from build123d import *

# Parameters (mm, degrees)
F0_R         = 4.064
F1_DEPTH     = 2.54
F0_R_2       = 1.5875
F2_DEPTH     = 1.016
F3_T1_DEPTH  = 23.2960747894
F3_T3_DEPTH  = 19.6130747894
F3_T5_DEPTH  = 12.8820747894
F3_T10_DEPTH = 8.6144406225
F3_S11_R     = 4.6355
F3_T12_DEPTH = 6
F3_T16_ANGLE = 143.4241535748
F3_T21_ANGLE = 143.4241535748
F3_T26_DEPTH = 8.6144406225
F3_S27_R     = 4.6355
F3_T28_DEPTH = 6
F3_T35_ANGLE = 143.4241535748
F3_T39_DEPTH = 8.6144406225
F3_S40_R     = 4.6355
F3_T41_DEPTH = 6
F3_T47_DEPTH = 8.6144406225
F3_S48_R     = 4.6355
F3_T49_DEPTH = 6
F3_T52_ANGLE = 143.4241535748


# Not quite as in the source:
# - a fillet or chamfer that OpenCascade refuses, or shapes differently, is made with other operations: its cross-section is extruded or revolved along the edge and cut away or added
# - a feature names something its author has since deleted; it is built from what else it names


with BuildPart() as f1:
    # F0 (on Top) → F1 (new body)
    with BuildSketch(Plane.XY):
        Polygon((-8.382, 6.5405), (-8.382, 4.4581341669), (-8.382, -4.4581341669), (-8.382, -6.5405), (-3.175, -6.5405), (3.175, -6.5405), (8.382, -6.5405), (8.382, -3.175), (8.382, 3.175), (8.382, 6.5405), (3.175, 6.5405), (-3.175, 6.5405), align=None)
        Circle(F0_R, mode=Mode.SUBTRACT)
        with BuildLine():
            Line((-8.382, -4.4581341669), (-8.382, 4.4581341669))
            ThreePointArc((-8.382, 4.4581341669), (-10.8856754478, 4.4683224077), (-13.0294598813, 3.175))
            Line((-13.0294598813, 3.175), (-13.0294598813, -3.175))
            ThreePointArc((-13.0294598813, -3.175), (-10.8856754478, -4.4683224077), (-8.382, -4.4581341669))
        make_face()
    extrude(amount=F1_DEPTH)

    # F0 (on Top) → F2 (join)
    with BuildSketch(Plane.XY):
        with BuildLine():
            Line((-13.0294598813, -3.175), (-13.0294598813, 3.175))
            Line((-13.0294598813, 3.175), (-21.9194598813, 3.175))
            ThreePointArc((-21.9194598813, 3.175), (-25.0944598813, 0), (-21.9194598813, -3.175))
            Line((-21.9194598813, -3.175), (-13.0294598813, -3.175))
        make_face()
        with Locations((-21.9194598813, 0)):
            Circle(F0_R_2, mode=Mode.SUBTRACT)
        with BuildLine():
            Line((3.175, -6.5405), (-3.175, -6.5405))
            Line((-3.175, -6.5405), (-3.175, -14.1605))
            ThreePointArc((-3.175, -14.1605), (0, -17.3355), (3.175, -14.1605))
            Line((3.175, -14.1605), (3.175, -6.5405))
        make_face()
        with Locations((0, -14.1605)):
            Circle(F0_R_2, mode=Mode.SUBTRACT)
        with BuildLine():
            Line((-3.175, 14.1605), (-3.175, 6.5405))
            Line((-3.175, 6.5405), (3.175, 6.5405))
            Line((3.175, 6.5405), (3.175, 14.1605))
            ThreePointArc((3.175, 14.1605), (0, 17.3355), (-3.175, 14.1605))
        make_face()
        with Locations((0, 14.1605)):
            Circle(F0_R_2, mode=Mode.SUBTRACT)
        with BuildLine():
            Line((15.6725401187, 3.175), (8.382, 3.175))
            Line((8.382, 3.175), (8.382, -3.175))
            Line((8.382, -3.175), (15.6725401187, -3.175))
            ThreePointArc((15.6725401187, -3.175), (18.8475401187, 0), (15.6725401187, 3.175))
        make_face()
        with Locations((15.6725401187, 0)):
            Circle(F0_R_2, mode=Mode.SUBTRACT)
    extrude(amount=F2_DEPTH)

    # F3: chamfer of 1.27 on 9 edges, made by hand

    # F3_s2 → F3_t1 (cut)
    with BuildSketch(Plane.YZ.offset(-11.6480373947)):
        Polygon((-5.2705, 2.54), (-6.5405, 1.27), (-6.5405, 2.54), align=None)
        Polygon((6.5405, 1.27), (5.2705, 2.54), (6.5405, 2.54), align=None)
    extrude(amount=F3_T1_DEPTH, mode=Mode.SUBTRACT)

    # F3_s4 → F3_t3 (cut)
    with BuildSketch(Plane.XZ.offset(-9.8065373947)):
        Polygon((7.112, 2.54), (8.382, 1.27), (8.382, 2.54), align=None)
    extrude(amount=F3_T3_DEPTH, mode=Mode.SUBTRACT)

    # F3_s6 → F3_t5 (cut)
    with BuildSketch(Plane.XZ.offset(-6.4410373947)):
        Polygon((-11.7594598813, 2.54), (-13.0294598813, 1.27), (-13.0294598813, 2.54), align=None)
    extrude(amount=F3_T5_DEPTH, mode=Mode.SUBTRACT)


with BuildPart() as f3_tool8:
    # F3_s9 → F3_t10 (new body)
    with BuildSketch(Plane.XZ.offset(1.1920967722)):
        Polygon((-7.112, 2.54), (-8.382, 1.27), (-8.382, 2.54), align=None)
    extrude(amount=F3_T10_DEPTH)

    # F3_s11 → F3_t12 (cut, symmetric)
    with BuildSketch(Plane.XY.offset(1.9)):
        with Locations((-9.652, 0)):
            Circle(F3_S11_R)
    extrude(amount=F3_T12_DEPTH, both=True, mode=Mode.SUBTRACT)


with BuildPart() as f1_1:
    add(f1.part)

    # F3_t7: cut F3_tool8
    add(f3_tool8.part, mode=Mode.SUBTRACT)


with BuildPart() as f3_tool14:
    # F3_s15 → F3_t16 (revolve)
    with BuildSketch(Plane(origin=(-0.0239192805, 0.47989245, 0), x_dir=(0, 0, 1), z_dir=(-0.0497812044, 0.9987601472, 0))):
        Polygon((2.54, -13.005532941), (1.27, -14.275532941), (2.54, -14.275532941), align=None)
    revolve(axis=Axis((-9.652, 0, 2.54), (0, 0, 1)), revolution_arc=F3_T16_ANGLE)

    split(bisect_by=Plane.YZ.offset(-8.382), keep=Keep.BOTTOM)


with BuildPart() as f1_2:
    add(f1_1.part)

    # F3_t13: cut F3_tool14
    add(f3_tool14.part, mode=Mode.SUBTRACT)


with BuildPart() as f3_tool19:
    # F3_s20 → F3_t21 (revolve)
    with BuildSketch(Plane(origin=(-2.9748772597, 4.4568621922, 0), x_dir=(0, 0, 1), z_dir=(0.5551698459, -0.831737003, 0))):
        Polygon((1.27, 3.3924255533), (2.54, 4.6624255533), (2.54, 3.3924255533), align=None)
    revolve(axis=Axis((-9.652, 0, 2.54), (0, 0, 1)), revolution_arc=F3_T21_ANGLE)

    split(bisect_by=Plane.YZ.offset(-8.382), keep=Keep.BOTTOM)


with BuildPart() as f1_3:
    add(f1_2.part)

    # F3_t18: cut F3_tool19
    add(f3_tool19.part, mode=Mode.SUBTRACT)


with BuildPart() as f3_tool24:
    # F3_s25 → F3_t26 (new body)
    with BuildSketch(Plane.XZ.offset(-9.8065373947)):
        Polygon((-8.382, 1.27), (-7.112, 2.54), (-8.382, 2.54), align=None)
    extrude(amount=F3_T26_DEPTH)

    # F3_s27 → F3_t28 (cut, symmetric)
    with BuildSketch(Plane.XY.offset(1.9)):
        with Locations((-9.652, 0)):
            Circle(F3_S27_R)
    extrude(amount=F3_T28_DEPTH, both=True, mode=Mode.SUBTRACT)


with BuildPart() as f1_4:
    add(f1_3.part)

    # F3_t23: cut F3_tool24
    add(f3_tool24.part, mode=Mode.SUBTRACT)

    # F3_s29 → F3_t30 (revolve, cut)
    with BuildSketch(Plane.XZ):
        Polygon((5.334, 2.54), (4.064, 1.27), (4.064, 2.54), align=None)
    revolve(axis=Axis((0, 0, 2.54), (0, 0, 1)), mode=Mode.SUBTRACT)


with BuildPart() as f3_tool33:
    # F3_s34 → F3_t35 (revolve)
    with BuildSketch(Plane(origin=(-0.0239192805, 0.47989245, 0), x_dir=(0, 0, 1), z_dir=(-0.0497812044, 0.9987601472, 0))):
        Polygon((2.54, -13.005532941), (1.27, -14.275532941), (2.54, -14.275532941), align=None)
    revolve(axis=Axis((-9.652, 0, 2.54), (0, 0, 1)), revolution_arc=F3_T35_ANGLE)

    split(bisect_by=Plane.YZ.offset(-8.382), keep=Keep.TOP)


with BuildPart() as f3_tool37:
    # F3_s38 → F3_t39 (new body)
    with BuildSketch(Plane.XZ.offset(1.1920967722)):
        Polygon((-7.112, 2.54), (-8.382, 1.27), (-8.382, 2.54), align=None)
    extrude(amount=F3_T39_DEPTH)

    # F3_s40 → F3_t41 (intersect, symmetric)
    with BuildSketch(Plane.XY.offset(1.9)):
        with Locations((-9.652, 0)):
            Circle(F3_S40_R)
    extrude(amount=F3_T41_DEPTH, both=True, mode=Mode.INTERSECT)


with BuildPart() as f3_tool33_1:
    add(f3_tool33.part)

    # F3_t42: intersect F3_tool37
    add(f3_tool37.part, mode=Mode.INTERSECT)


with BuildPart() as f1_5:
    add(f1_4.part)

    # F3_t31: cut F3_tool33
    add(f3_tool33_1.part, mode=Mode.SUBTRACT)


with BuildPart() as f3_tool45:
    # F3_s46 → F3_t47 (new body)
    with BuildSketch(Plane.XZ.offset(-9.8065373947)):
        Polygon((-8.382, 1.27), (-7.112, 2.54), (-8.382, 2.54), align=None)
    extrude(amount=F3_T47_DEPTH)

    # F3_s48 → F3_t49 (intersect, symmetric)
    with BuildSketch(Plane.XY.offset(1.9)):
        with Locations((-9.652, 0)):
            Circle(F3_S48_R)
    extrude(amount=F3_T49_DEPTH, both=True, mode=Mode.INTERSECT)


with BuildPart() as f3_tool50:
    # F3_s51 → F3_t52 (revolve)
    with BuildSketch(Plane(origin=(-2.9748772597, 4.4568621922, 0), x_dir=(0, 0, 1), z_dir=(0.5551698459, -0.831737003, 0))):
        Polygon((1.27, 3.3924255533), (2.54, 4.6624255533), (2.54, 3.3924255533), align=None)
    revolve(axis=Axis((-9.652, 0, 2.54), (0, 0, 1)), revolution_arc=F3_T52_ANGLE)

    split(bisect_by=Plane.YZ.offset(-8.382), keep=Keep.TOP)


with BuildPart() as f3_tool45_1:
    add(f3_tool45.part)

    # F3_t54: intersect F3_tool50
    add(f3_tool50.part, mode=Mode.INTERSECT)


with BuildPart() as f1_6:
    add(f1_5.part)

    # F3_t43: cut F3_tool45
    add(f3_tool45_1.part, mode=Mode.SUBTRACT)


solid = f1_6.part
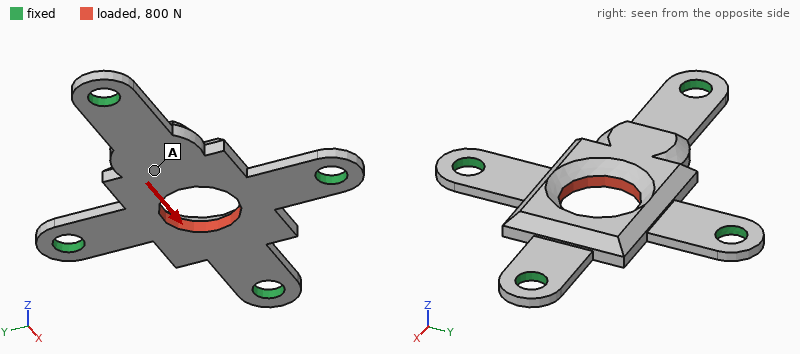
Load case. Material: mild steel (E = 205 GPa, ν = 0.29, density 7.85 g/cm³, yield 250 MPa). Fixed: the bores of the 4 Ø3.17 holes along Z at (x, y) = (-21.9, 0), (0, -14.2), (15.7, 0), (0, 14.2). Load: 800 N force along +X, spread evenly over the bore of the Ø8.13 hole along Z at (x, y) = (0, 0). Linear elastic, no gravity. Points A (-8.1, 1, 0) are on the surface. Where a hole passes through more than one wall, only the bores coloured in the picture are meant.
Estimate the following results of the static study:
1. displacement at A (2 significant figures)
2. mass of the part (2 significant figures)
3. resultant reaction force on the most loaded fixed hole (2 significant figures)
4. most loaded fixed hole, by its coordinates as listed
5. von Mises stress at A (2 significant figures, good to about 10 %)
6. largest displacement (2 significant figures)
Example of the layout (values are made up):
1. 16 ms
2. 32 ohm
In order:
1. 2.7 µm
2. 5.4 g
3. 350 N
4. (15.7, 0)
5. 32 MPa
6. 3.5 µm
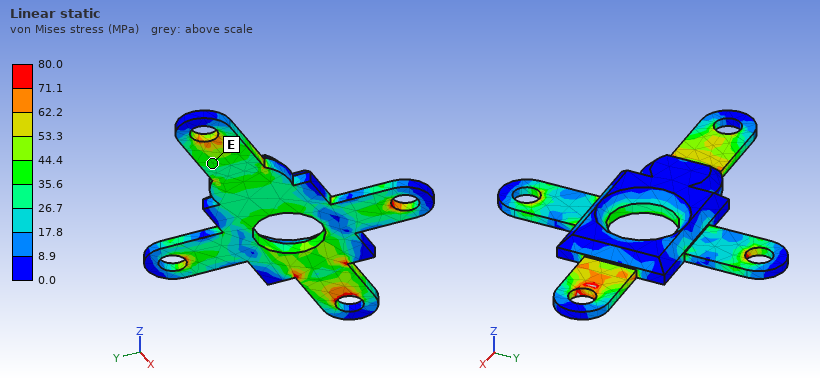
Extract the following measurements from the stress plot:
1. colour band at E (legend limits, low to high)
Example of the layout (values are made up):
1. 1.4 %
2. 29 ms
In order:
1. 35.6 to 44.4 MPa
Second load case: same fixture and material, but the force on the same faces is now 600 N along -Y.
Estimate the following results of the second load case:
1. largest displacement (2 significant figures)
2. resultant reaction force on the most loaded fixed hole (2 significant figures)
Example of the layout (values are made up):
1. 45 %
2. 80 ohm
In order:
1. 2.4 µm
2. 260 N
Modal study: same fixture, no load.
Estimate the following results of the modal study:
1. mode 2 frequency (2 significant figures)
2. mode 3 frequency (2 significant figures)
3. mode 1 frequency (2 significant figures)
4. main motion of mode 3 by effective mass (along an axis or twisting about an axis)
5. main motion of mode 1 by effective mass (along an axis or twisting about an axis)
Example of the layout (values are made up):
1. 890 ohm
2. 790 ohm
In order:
1. 14 kHz
2. 16 kHz
3. 8200 Hz
4. twisting about X
5. along Z
